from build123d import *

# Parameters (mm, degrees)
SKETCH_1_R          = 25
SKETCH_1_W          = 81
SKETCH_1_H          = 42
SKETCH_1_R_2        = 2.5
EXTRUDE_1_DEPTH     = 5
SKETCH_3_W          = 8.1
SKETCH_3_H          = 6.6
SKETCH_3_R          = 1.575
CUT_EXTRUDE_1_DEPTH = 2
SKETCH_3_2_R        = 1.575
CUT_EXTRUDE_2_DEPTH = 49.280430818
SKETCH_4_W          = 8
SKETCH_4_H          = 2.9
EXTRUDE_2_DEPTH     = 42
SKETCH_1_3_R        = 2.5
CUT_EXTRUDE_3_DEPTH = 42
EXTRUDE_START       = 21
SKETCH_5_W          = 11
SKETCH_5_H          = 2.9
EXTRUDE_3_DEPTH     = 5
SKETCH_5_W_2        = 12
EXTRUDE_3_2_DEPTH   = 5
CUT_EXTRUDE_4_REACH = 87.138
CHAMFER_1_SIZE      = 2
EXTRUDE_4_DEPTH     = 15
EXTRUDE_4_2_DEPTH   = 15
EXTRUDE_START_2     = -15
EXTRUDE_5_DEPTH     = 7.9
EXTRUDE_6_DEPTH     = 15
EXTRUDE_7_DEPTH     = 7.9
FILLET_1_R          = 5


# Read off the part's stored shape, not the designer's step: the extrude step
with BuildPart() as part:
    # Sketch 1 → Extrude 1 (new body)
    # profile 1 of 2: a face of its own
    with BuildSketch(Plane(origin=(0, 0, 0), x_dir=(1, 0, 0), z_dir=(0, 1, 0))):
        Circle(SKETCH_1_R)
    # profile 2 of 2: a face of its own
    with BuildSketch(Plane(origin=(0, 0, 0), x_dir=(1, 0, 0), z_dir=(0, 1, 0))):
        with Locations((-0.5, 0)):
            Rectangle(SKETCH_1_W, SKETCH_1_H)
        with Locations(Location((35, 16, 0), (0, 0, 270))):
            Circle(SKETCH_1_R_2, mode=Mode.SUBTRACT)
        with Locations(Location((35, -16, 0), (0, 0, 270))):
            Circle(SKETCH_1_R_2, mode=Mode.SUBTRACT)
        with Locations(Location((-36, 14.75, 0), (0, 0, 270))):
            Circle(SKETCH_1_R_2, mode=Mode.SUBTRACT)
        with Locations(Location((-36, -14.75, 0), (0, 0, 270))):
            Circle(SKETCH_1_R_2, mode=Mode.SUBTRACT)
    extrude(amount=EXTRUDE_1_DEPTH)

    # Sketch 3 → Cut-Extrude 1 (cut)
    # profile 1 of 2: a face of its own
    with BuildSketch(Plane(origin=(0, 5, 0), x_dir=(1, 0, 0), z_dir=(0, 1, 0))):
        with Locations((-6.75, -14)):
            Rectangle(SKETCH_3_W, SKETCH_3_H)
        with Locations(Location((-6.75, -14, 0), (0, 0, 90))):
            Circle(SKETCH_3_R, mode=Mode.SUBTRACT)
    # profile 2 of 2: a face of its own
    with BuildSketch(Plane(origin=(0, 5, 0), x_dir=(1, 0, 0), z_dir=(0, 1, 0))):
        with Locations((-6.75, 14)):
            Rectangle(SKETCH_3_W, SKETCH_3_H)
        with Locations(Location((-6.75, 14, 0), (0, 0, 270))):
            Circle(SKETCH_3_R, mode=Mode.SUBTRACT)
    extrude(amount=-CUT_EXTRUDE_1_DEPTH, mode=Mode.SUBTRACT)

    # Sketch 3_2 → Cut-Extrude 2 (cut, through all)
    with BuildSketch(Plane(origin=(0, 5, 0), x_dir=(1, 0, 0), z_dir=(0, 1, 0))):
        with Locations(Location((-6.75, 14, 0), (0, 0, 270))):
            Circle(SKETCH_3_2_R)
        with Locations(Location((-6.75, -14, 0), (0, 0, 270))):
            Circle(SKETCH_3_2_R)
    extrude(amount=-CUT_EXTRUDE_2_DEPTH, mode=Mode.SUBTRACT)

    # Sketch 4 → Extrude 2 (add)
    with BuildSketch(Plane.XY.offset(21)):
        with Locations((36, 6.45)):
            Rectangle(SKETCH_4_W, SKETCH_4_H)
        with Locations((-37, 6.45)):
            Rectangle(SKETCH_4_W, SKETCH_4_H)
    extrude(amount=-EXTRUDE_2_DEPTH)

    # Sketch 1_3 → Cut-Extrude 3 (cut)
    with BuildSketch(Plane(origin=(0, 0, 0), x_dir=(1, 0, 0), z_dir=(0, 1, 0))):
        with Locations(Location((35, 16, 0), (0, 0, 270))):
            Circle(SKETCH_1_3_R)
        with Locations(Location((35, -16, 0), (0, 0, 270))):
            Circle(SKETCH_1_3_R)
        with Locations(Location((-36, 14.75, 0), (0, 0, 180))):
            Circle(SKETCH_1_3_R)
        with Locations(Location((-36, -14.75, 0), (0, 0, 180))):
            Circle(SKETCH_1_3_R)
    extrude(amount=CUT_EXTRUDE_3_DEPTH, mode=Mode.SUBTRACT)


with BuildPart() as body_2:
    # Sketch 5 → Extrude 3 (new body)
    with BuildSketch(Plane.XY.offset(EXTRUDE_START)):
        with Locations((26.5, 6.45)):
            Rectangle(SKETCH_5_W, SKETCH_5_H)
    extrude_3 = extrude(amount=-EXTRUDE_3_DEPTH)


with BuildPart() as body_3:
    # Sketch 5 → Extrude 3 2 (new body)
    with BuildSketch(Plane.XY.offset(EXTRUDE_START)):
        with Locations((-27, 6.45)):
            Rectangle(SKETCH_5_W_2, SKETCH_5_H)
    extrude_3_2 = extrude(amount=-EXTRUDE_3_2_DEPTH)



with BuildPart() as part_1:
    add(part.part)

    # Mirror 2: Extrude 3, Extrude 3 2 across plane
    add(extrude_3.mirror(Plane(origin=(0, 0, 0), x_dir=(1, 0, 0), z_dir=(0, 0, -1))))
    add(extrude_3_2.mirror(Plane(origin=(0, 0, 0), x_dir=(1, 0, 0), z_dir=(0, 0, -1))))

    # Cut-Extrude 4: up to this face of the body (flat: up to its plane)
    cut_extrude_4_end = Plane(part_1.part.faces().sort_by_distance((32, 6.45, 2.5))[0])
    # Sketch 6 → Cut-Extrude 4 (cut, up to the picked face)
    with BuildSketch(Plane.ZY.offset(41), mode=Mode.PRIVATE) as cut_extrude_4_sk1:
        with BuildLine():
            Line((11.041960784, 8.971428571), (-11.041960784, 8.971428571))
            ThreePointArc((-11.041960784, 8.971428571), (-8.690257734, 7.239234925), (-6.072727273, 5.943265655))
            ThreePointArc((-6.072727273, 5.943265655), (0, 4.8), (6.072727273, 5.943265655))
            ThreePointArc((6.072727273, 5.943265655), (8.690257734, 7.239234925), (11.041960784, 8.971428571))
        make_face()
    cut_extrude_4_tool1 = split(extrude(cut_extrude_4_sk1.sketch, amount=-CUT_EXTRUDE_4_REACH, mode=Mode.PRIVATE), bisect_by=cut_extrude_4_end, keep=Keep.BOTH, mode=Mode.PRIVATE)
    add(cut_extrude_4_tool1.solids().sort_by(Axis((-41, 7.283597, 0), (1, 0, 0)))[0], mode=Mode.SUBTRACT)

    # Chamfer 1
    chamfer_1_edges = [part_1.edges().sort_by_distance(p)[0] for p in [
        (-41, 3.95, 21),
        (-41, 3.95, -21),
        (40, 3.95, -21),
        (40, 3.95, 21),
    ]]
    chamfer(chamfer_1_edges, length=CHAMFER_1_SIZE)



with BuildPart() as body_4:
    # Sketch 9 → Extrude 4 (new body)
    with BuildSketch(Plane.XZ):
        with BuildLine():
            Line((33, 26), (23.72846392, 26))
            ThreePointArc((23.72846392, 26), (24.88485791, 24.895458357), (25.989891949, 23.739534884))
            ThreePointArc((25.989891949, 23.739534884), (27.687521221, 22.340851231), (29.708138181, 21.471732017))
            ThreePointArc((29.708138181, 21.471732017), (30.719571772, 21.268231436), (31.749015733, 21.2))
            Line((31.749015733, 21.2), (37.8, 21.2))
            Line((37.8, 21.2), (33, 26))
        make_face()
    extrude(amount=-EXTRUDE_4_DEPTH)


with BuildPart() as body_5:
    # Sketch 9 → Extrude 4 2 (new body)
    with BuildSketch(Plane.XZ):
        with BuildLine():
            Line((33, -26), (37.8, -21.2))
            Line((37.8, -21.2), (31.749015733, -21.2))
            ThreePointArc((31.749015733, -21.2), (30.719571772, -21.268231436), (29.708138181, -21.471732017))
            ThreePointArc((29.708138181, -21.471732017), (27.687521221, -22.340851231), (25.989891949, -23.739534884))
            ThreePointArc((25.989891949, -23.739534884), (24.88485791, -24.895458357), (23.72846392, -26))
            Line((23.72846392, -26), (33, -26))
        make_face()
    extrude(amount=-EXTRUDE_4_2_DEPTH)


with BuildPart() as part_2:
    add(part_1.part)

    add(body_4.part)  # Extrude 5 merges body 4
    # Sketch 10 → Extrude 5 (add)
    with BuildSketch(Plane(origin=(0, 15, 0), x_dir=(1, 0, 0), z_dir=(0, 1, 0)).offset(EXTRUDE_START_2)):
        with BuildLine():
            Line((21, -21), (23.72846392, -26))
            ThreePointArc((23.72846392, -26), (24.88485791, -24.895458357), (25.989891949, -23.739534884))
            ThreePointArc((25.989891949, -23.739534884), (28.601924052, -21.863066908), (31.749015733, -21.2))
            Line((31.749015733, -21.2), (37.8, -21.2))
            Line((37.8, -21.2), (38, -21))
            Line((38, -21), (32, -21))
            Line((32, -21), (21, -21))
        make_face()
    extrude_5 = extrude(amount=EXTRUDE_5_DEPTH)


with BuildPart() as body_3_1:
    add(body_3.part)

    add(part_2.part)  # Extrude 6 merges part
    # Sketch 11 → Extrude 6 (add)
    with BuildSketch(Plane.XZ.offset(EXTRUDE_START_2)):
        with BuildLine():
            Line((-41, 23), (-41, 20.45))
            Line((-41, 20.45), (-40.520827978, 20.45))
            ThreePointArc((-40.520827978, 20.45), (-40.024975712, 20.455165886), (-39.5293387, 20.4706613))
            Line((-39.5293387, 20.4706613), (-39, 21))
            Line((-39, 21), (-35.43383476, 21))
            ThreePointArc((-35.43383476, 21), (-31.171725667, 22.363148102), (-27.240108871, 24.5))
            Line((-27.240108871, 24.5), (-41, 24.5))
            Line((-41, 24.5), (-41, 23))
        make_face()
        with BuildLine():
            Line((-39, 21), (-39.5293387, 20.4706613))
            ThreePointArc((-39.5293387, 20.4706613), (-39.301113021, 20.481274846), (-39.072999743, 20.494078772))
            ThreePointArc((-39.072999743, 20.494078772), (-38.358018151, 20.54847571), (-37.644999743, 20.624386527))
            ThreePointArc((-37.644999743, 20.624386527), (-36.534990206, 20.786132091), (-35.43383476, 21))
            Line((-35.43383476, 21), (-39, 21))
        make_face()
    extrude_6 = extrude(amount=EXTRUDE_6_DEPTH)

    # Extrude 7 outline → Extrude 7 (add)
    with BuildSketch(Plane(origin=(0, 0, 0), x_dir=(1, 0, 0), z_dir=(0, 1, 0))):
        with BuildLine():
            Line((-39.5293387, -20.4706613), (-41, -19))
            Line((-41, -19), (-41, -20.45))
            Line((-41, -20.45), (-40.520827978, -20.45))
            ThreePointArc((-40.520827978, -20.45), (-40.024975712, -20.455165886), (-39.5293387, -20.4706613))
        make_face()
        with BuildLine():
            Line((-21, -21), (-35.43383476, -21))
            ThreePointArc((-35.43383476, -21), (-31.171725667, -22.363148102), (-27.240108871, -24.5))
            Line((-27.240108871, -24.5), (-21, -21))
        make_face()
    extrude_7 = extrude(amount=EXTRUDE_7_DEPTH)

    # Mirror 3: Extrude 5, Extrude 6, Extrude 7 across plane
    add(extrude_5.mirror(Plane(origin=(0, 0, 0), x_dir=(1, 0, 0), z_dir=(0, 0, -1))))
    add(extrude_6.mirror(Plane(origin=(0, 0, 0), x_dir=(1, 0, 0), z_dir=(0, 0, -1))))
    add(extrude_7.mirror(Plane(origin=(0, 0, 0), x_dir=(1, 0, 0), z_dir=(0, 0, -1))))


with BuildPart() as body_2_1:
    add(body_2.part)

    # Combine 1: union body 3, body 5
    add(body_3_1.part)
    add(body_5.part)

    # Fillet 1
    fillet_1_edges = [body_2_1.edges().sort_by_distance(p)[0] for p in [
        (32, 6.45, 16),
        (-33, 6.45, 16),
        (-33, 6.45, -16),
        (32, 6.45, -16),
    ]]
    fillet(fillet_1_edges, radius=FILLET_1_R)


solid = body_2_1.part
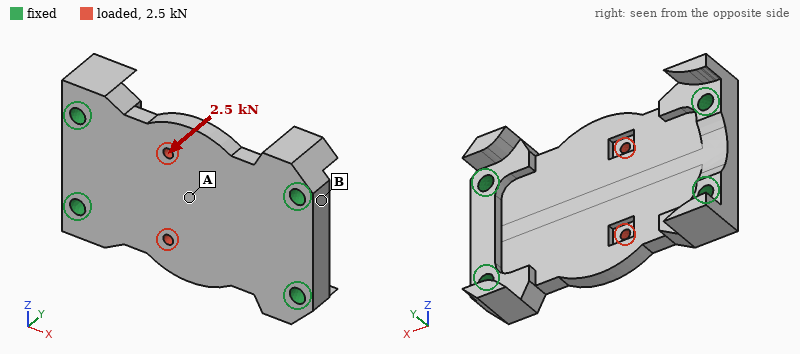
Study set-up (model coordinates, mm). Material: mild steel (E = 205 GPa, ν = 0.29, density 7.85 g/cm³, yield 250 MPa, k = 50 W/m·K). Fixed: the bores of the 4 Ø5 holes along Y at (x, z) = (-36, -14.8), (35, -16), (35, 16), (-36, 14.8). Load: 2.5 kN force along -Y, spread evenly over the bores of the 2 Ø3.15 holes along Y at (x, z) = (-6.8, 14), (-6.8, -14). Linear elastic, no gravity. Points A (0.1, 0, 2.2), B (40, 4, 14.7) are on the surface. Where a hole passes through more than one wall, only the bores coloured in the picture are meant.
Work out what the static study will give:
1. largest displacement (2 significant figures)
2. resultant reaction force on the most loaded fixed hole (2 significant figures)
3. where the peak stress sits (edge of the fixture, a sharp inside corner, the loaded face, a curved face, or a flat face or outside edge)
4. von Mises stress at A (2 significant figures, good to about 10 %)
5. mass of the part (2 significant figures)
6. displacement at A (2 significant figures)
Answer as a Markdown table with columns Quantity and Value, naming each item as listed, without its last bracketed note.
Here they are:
| Quantity | Value |
|---|---|
| largest displacement | 37 µm |
| resultant reaction force on the most loaded fixed hole | 960 N |
| where the peak stress sits | the loaded face |
| von Mises stress at A | 59 MPa |
| mass of the part | 170 g |
| displacement at A | 30 µm |
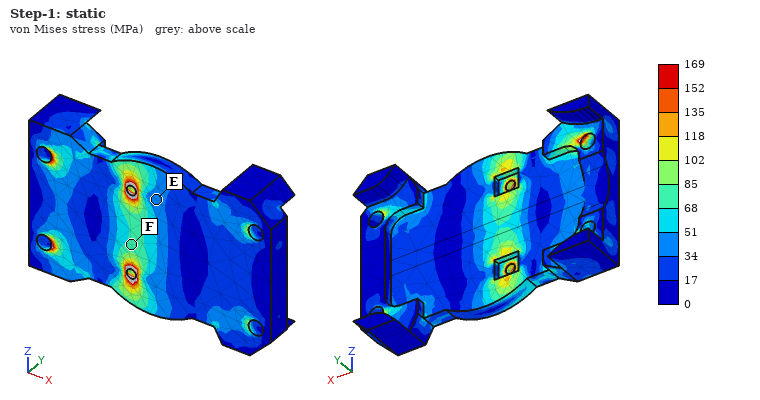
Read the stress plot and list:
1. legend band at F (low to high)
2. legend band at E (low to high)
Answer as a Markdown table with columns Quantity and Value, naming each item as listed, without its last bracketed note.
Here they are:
| Quantity | Value |
|---|---|
| legend band at F | 68 to 85 MPa |
| legend band at E | 34 to 51 MPa |
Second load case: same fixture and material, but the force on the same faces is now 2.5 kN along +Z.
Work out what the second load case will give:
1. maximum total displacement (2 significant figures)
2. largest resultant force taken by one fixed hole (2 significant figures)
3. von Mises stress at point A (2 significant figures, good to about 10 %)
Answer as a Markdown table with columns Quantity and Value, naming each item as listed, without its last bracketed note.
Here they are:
| Quantity | Value |
|---|---|
| maximum total displacement | 4.2 µm |
| largest resultant force taken by one fixed hole | 980 N |
| von Mises stress at point A | 9.1 MPa |
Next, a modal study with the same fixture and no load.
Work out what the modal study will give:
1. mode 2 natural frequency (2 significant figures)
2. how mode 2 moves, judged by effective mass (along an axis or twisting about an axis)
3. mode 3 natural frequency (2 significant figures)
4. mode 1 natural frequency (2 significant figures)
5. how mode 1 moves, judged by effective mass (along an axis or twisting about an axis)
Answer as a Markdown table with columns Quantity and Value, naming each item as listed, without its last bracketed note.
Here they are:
| Quantity | Value |
|---|---|
| mode 2 natural frequency | 8600 Hz |
| how mode 2 moves, judged by effective mass | twisting about X |
| mode 3 natural frequency | 15 kHz |
| mode 1 natural frequency | 6300 Hz |
| how mode 1 moves, judged by effective mass | along Y |
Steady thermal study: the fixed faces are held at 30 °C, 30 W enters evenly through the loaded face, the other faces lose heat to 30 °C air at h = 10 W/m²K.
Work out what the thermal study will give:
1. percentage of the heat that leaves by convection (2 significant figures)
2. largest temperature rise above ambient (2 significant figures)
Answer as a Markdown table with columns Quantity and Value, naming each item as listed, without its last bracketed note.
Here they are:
| Quantity | Value |
|---|---|
| percentage of the heat that leaves by convection | 5.6 % |
| largest temperature rise above ambient | 61 K |
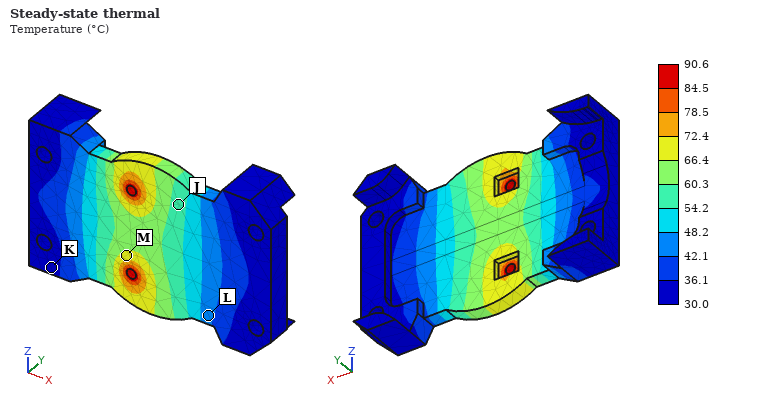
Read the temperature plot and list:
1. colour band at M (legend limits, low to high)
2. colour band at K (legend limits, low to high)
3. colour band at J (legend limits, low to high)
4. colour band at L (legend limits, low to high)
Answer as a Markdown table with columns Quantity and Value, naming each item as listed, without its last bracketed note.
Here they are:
| Quantity | Value |
|---|---|
| colour band at M | 66.4 to 72.4 °C |
| colour band at K | 30.0 to 36.1 °C |
| colour band at J | 54.2 to 60.3 °C |
| colour band at L | 42.1 to 48.2 °C |
